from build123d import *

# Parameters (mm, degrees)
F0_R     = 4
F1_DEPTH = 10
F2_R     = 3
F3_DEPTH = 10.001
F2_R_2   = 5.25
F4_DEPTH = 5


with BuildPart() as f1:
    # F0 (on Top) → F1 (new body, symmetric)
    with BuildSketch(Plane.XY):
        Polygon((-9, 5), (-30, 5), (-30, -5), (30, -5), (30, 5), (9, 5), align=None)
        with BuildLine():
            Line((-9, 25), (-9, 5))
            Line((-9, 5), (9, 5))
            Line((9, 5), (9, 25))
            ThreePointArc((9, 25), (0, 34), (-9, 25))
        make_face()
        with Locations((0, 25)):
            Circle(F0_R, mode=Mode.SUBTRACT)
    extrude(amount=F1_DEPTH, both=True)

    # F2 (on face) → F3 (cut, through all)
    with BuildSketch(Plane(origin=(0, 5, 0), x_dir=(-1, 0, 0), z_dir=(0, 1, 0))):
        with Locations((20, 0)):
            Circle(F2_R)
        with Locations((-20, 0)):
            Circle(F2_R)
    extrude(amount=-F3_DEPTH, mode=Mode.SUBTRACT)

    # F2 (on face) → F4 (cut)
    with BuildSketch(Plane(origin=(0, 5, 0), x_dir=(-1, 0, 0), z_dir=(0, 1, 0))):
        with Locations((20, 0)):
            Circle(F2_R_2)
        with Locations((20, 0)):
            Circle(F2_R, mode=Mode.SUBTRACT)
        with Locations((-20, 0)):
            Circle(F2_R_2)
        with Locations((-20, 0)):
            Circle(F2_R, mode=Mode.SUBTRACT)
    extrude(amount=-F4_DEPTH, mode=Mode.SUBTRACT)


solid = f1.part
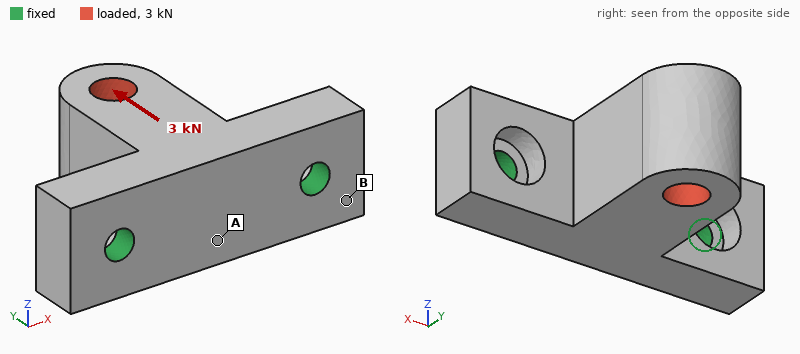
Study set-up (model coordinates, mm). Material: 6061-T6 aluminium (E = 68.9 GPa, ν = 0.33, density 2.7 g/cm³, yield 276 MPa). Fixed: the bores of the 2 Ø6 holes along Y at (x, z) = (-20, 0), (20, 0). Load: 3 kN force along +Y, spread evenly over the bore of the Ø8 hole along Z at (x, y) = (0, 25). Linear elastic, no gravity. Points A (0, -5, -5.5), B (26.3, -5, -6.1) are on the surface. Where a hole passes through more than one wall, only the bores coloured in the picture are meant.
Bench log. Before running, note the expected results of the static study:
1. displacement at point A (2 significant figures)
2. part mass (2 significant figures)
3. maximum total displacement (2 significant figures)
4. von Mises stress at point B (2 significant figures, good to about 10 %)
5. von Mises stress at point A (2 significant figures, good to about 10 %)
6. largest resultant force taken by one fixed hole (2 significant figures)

11 µm
53 g
15 µm
6.6 MPa
15 MPa
1.8 kN
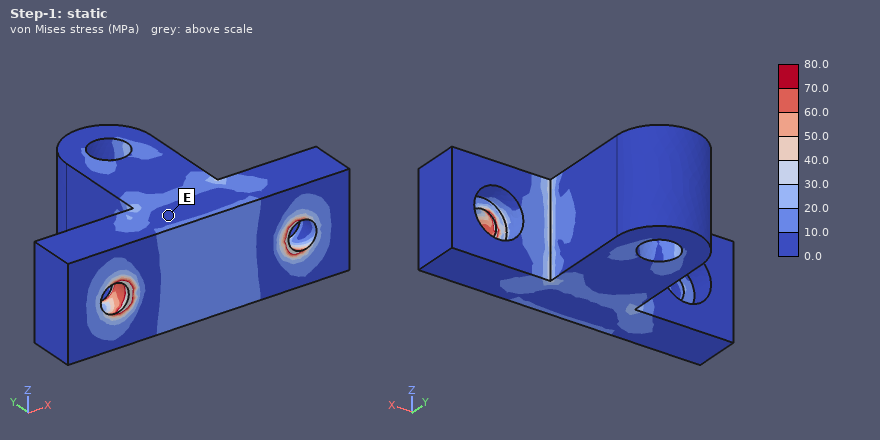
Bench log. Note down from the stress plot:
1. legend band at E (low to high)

0.0 to 10.0 MPa
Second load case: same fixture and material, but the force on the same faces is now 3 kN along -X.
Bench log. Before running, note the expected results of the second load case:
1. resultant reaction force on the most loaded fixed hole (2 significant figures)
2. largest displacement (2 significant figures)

2.8 kN
71 µm
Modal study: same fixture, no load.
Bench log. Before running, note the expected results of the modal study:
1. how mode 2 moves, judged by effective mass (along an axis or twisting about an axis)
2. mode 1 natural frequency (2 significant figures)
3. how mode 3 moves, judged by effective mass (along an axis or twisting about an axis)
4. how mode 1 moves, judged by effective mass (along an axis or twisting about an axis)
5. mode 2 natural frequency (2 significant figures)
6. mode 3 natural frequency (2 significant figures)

along X
4400 Hz
along Y
along Z
10 kHz
13 kHz
